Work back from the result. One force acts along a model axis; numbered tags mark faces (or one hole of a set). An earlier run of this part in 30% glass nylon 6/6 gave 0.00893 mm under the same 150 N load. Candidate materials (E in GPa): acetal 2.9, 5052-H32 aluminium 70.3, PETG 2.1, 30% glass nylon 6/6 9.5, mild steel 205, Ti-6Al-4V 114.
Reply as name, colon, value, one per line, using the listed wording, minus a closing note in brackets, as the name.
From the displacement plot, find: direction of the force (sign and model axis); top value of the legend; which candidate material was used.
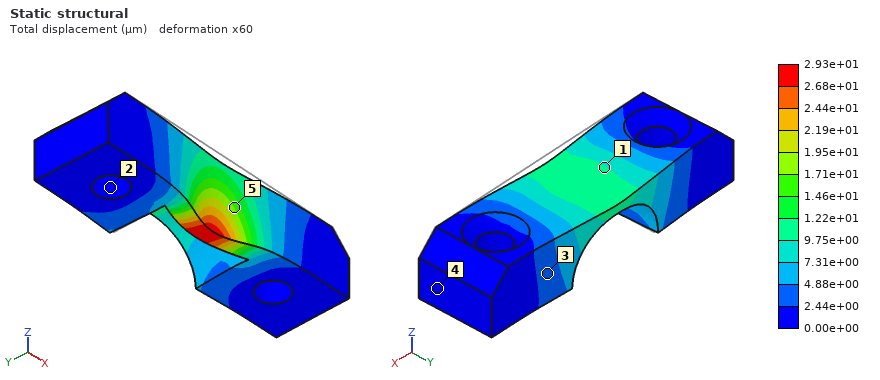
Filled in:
direction of the force: +Y
top value of the legend: 2.93e+01 µm
which candidate material was used: acetal
